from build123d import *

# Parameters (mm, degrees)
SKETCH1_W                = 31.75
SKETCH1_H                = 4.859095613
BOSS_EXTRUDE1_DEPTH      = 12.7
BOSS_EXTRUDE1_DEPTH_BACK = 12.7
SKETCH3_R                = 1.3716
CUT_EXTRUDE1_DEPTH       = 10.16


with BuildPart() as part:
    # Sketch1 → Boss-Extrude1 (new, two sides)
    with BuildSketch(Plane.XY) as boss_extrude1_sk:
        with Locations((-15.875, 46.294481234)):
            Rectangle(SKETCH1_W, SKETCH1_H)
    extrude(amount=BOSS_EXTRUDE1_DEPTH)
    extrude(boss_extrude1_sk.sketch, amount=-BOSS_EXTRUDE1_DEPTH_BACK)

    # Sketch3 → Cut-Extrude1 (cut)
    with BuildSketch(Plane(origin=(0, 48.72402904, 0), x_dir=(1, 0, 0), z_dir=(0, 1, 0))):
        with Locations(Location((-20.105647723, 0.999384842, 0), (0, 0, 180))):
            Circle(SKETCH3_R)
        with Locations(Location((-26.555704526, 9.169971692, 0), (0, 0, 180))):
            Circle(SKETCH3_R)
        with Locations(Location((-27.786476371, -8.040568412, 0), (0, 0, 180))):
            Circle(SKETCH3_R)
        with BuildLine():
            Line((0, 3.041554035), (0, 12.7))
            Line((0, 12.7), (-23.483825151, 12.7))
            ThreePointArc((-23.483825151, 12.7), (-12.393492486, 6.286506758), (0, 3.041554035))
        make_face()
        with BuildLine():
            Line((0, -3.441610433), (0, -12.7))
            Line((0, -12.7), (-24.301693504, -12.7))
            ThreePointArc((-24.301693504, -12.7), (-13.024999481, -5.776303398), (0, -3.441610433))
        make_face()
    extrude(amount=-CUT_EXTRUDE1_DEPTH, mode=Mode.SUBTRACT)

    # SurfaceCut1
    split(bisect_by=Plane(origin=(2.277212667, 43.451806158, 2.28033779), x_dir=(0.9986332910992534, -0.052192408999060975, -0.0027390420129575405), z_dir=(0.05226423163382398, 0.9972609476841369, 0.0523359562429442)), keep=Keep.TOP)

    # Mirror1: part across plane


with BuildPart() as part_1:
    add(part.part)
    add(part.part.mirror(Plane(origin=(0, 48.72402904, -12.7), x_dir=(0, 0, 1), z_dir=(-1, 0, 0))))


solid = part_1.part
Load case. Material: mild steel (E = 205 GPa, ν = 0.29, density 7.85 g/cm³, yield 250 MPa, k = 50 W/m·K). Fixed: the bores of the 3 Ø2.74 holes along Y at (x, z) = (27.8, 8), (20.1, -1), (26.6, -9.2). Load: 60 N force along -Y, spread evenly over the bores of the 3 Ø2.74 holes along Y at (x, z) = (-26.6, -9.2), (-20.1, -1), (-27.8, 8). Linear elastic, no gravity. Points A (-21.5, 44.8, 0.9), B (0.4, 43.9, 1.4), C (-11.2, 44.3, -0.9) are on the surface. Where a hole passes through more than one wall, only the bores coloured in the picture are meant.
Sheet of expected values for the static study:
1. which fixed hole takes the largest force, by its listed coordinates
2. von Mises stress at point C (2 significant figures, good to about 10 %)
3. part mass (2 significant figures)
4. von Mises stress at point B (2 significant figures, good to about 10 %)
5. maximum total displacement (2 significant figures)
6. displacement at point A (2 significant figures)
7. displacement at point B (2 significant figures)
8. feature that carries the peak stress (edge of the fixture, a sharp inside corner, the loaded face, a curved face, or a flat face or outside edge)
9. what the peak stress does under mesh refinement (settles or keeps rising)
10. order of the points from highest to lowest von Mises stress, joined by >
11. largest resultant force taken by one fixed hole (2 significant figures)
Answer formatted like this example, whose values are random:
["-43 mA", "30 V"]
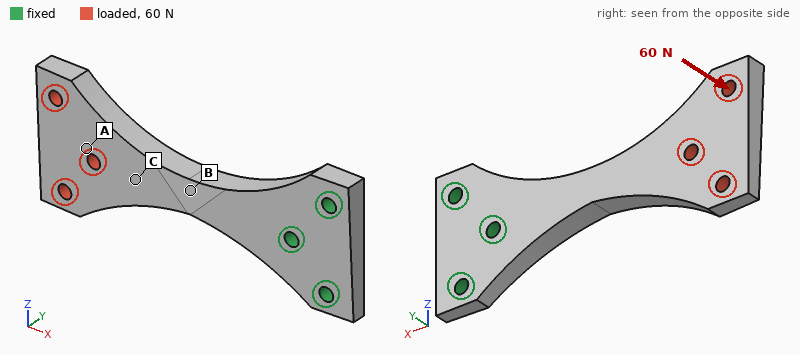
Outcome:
["(20.1, -1)", "23 MPa", "31 g", "57 MPa", "0.15 mm", "0.10 mm", "0.029 mm", "edge of the fixture", "keeps rising", "B > C > A", "200 N"]
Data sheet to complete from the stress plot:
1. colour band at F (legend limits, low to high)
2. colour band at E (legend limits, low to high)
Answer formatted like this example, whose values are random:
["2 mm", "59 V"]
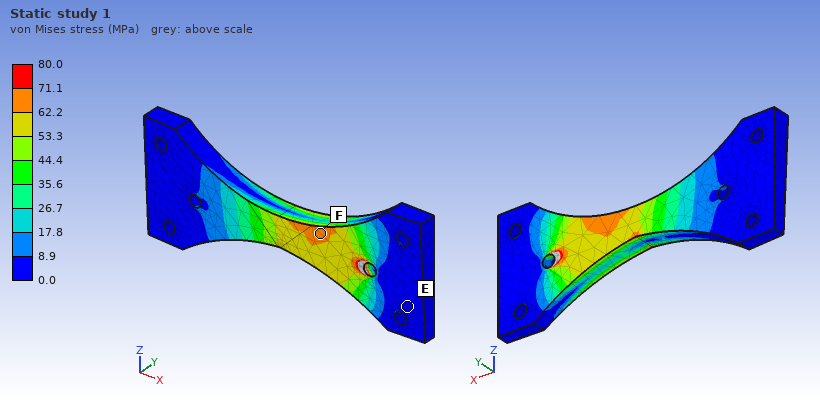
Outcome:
["62.2 to 71.1 MPa", "0.0 to 8.9 MPa"]
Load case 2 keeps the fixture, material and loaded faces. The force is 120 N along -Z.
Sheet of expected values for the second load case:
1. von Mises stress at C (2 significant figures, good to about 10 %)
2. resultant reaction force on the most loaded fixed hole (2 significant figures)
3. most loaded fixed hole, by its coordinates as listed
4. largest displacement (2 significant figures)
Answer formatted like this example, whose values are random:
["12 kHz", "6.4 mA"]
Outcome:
["13 MPa", "310 N", "(27.8, 8)", "82 µm"]
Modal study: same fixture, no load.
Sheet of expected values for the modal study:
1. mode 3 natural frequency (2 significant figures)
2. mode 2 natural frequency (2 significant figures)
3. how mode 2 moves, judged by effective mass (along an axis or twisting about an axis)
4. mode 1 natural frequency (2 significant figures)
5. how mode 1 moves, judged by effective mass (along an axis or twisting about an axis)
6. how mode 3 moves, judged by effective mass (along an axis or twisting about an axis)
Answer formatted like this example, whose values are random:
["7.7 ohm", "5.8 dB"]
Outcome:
["4500 Hz", "2100 Hz", "along Z", "1100 Hz", "along Y", "twisting about X"]
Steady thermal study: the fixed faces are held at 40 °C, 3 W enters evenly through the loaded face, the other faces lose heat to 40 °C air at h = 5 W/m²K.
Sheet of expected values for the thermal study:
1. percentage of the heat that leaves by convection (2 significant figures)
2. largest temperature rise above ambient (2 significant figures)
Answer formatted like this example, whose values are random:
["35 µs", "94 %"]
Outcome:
["12 %", "55 K"]
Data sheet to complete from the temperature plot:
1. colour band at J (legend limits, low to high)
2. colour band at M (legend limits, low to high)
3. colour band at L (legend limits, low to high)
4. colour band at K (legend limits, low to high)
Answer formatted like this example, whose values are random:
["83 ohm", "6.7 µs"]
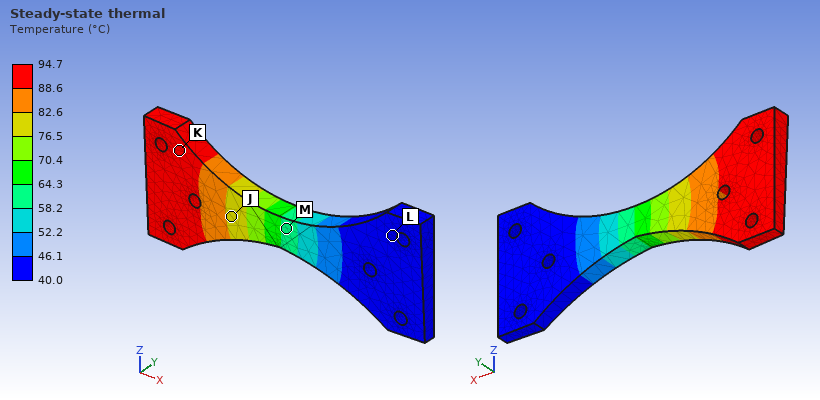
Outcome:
["76.5 to 82.6 °C", "58.2 to 64.3 °C", "40.0 to 46.1 °C", "88.6 to 94.7 °C"]
